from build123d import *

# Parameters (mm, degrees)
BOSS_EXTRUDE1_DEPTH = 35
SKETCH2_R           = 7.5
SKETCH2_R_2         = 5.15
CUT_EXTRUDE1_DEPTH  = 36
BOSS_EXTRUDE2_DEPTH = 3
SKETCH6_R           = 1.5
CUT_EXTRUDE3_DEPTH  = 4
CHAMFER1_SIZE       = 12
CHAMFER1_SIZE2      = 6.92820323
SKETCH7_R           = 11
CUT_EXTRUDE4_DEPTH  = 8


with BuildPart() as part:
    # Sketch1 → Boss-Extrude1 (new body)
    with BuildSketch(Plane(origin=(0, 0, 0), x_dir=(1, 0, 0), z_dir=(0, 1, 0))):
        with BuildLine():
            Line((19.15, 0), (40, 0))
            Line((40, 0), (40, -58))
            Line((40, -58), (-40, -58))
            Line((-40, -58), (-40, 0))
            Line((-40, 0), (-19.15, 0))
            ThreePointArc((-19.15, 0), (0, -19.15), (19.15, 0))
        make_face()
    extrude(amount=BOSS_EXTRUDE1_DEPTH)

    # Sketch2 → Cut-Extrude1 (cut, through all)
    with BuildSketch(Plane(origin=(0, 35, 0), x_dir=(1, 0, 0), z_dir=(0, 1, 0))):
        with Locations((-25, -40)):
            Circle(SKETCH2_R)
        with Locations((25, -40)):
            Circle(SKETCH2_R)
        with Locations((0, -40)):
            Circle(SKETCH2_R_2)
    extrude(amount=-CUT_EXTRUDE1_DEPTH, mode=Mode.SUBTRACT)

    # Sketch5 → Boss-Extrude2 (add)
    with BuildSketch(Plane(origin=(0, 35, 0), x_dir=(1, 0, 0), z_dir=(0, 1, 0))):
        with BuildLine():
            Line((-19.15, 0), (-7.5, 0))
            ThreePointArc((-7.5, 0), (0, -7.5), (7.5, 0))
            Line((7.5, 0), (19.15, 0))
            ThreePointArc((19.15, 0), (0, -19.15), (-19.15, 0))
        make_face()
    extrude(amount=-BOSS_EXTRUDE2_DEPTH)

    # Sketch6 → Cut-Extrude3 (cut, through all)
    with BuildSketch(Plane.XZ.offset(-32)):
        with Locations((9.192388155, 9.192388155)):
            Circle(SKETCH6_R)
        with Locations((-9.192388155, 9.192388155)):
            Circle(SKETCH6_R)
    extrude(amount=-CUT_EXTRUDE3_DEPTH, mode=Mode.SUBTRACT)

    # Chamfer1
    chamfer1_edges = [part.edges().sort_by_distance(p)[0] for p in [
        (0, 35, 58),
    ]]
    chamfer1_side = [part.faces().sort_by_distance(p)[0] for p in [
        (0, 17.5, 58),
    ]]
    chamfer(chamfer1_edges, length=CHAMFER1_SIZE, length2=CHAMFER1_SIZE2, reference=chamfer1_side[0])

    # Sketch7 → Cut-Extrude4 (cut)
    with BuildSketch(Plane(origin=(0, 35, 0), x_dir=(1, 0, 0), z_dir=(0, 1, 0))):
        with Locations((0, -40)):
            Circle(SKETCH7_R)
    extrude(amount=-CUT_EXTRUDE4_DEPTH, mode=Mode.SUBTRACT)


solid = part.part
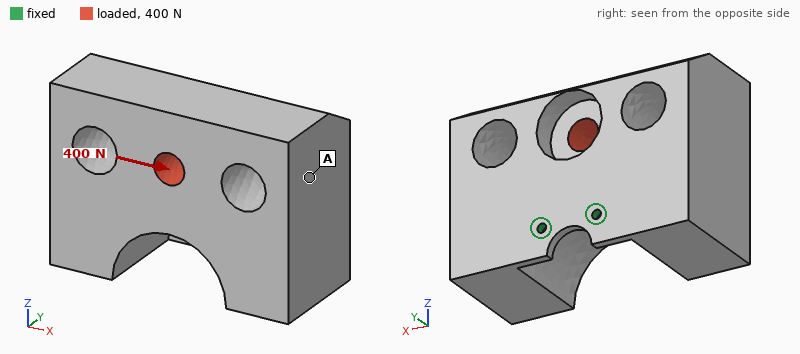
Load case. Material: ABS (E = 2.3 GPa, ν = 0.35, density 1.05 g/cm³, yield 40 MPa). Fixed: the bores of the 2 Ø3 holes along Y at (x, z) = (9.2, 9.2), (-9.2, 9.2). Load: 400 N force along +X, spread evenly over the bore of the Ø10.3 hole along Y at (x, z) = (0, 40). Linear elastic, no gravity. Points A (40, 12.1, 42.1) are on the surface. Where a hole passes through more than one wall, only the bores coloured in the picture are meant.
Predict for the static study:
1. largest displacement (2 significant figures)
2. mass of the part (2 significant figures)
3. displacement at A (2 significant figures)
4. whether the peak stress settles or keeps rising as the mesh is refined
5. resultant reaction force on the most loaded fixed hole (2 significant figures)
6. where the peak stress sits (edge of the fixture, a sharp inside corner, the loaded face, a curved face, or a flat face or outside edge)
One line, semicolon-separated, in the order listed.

1.2 mm; 130 g; 0.98 mm; keeps rising; 720 N; edge of the fixture
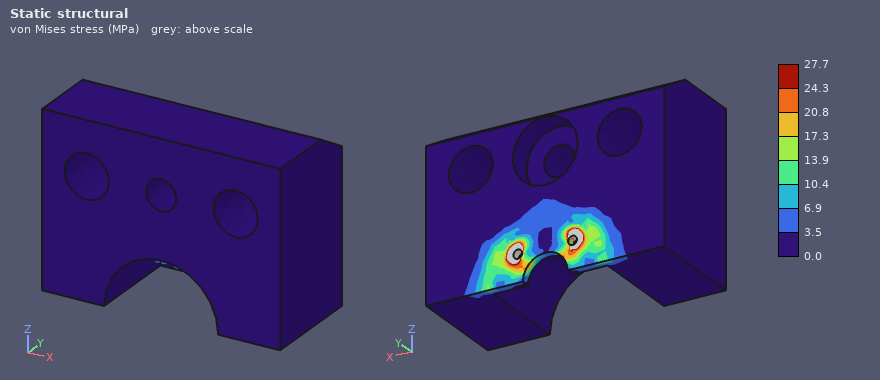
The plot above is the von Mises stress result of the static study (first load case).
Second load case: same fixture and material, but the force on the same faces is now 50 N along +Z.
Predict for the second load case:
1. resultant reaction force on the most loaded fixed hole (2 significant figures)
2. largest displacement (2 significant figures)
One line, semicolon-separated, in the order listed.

27 N; 1.1 mm
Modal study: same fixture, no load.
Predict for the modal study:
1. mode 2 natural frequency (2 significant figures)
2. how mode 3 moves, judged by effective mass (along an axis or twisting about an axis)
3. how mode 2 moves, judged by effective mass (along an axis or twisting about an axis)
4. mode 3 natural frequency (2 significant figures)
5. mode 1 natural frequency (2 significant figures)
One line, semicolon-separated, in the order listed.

290 Hz; along X; along X; 460 Hz; 100 Hz
